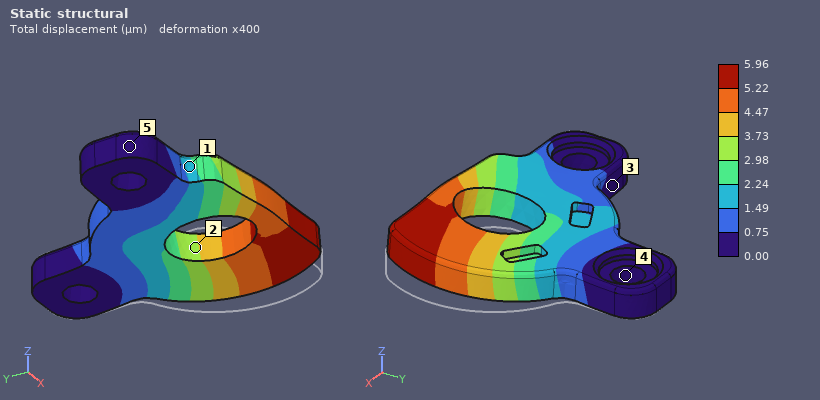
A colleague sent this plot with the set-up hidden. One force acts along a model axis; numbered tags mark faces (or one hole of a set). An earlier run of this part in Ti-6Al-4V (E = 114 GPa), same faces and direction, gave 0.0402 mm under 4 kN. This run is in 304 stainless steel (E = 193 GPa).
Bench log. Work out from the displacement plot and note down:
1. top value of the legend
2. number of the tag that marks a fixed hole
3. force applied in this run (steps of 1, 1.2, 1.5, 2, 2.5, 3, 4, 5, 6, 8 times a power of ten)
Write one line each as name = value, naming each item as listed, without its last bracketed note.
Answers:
top value of the legend = 5.96 µm
number of the tag that marks a fixed hole = 4
force applied in this run = 1 kN
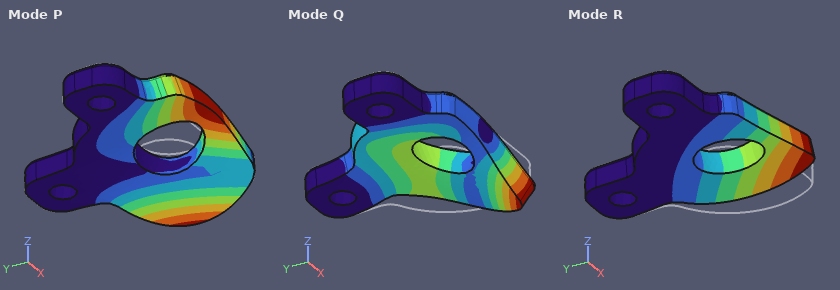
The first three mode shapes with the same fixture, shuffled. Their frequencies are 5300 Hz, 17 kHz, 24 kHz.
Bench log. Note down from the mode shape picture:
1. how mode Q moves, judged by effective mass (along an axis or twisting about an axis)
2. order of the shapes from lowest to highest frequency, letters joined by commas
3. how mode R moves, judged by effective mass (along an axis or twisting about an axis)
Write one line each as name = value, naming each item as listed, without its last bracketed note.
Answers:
how mode Q moves, judged by effective mass = along Z
order of the shapes from lowest to highest frequency, letters joined by commas = R, P, Q
how mode R moves, judged by effective mass = along Z
